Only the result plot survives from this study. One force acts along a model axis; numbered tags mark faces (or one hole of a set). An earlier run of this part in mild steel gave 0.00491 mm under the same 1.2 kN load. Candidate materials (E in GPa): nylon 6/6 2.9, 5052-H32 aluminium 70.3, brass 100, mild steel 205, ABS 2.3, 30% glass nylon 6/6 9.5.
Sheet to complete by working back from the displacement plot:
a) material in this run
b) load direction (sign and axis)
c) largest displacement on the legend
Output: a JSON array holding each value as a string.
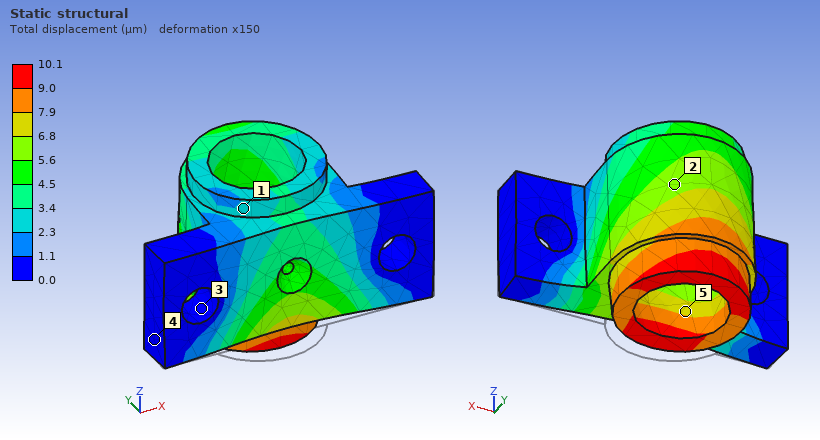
["brass", "+Y", "10.1 µm"]
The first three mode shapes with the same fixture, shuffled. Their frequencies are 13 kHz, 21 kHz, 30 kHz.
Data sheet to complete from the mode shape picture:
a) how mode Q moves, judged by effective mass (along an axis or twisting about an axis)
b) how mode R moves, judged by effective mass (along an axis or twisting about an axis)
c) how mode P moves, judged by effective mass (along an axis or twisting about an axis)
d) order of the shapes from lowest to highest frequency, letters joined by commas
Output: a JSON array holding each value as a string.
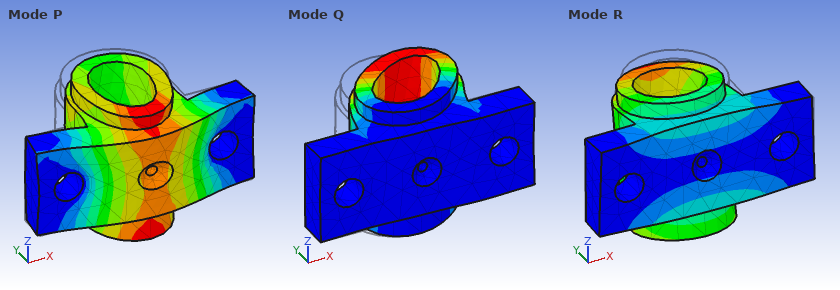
["along X", "along Z", "along Y", "R, Q, P"]
